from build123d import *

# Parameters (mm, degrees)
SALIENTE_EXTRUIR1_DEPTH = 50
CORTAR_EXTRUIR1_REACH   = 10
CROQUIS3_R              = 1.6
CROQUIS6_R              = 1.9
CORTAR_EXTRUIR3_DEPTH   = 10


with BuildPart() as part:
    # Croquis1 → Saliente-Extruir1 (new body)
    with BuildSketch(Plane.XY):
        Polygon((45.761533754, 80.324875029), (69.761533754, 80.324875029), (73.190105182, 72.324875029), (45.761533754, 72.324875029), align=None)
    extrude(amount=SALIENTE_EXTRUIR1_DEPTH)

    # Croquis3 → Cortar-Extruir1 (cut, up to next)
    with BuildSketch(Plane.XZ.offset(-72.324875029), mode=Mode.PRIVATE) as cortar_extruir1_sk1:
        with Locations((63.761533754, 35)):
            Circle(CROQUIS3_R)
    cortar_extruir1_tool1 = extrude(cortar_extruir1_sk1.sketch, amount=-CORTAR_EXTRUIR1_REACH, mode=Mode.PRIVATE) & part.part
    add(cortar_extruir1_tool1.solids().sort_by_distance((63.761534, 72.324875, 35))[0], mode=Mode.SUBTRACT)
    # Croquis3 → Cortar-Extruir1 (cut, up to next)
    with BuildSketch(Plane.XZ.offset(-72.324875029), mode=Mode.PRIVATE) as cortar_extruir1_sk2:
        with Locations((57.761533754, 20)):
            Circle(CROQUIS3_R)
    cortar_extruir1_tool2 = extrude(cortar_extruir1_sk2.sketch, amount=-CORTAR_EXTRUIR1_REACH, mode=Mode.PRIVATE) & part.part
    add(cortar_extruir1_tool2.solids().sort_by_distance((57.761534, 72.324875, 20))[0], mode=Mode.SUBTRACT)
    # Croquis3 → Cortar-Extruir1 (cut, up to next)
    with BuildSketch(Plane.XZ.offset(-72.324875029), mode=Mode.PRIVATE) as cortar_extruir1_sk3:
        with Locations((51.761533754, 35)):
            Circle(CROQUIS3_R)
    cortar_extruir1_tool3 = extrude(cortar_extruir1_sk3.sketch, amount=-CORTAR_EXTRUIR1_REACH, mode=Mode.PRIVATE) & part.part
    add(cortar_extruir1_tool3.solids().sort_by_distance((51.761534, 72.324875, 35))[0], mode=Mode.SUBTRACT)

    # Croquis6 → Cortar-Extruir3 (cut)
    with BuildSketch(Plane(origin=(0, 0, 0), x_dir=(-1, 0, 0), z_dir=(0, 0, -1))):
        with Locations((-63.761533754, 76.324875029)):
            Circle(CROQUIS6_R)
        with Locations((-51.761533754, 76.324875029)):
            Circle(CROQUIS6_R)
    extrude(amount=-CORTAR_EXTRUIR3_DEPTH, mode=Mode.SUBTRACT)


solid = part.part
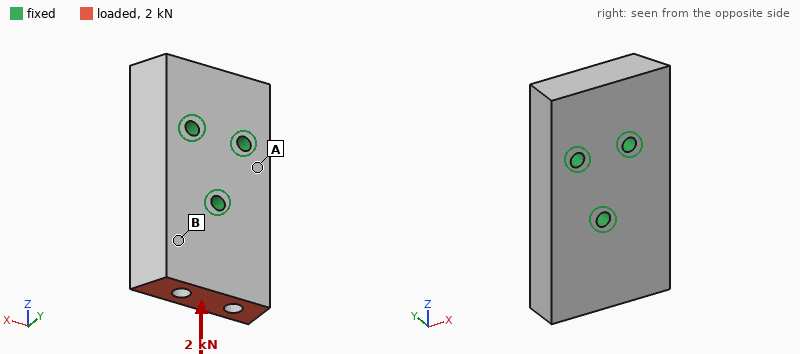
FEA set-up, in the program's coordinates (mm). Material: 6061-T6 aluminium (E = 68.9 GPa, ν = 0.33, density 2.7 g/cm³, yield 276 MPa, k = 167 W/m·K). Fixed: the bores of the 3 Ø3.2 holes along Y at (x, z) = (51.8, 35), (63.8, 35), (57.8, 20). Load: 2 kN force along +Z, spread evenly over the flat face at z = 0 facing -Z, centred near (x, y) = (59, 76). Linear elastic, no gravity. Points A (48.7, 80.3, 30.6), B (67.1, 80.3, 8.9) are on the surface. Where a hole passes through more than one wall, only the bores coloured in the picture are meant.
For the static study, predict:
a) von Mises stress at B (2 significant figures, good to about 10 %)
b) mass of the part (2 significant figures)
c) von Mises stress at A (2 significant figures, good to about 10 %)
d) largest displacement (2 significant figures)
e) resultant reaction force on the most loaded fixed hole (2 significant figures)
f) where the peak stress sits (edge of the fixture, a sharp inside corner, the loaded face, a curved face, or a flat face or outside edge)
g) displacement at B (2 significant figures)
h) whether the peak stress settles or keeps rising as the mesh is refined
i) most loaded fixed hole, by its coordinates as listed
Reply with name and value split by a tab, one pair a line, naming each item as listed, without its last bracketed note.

von Mises stress at B	10 MPa
mass of the part	27 g
von Mises stress at A	4.1 MPa
largest displacement	4.8 µm
resultant reaction force on the most loaded fixed hole	1.3 kN
where the peak stress sits	edge of the fixture
displacement at B	2.9 µm
whether the peak stress settles or keeps rising as the mesh is refined	keeps rising
most loaded fixed hole, by its coordinates as listed	(57.8, 20)
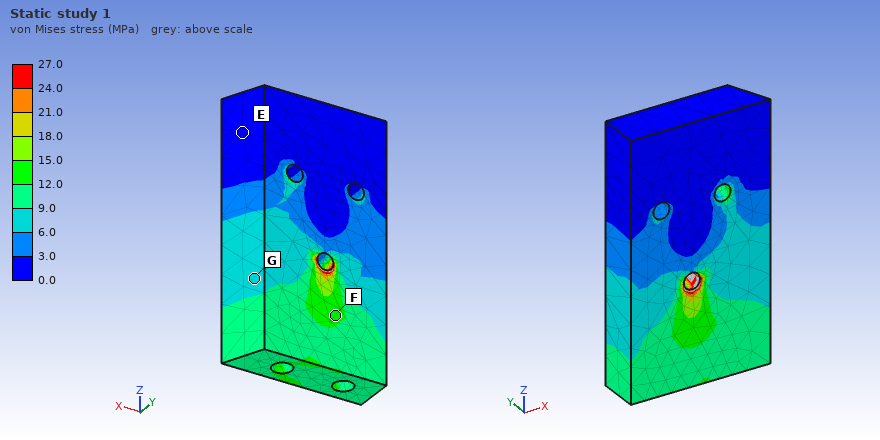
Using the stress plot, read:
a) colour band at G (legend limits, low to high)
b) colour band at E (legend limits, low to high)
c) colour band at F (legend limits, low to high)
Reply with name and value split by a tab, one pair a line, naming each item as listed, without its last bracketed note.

colour band at G	6.0 to 9.0 MPa
colour band at E	0.0 to 3.0 MPa
colour band at F	12.0 to 15.0 MPa
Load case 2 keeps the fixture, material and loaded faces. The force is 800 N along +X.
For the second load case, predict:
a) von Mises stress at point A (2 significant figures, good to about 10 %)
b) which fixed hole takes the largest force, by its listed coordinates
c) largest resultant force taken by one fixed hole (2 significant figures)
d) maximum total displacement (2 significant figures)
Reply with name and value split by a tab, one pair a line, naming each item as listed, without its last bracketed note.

von Mises stress at point A	9.9 MPa
which fixed hole takes the largest force, by its listed coordinates	(57.8, 20)
largest resultant force taken by one fixed hole	1.3 kN
maximum total displacement	15 µm
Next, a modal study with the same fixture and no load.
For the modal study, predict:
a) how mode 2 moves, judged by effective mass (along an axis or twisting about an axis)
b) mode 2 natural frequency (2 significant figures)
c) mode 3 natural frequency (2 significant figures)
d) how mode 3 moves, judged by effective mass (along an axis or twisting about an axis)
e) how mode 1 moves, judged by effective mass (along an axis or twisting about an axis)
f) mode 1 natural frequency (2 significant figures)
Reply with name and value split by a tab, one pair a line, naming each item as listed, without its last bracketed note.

how mode 2 moves, judged by effective mass	twisting about Z
mode 2 natural frequency	18 kHz
mode 3 natural frequency	20 kHz
how mode 3 moves, judged by effective mass	along X
how mode 1 moves, judged by effective mass	along Y
mode 1 natural frequency	13 kHz
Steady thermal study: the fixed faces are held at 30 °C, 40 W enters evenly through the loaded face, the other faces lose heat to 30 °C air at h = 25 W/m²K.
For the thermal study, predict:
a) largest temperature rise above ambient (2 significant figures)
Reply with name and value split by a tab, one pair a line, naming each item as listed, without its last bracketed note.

largest temperature rise above ambient	28 K
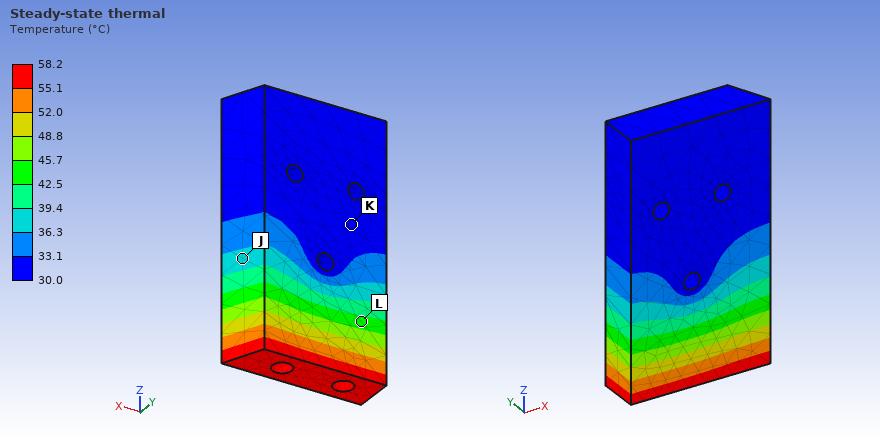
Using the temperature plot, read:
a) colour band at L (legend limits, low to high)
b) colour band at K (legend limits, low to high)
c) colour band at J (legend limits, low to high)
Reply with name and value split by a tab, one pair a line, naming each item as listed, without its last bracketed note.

colour band at L	42.5 to 45.7 °C
colour band at K	30.0 to 33.1 °C
colour band at J	36.3 to 39.4 °C
